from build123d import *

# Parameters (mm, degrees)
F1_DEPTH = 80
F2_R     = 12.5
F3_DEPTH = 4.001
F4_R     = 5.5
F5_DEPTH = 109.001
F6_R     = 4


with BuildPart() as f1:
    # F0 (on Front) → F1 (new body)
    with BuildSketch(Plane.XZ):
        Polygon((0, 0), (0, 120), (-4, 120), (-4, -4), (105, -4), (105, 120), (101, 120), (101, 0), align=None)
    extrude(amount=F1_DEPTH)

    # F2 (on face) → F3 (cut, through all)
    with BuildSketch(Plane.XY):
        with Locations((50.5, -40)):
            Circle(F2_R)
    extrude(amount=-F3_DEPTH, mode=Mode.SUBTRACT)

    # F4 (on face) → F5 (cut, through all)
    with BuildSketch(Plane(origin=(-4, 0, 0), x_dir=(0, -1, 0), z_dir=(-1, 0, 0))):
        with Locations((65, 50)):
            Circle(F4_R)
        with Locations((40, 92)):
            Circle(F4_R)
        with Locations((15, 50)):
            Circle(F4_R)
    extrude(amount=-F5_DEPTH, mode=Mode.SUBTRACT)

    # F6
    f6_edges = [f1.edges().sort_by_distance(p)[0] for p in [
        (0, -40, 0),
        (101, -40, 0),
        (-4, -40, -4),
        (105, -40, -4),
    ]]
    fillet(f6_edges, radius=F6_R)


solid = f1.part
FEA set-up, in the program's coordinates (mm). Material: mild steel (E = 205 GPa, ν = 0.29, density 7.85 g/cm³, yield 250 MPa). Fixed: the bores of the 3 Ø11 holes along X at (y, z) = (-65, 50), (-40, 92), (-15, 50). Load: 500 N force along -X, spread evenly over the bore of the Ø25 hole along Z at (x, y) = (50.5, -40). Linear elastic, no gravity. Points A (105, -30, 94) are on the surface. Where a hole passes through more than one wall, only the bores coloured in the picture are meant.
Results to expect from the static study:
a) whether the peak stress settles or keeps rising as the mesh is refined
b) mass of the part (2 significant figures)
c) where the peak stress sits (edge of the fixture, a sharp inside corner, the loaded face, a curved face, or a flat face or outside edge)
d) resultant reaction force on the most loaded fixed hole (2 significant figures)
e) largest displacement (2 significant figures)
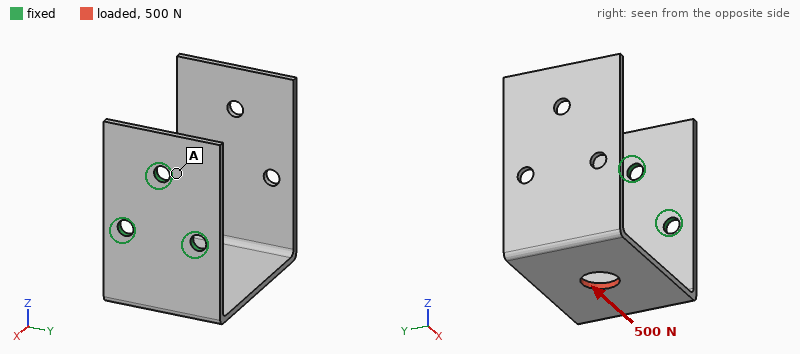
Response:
keeps rising
840 g
edge of the fixture
280 N
0.92 mm
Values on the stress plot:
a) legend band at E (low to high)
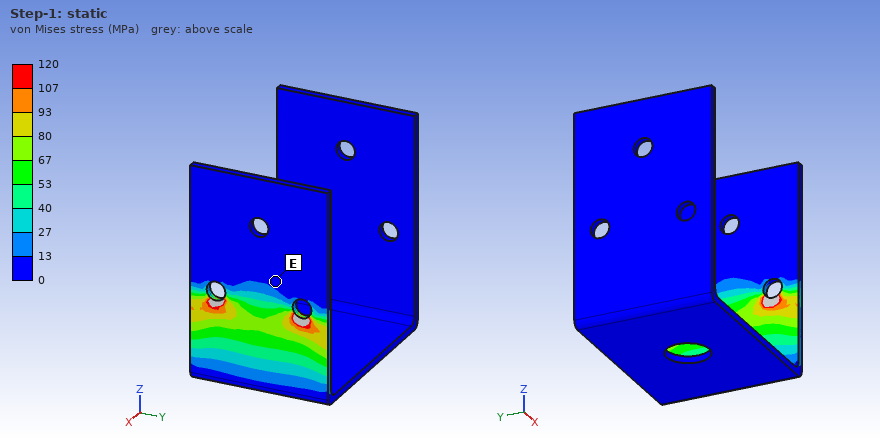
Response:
0 to 13 MPa
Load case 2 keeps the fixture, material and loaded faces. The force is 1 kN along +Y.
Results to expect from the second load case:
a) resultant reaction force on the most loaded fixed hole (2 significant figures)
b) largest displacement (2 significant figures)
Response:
1.3 kN
1.4 mm
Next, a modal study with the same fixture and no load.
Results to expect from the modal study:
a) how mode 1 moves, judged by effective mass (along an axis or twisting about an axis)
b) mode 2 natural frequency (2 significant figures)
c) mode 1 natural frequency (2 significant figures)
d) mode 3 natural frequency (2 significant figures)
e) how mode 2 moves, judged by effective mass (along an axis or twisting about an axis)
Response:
along Z
120 Hz
68 Hz
180 Hz
along Y
